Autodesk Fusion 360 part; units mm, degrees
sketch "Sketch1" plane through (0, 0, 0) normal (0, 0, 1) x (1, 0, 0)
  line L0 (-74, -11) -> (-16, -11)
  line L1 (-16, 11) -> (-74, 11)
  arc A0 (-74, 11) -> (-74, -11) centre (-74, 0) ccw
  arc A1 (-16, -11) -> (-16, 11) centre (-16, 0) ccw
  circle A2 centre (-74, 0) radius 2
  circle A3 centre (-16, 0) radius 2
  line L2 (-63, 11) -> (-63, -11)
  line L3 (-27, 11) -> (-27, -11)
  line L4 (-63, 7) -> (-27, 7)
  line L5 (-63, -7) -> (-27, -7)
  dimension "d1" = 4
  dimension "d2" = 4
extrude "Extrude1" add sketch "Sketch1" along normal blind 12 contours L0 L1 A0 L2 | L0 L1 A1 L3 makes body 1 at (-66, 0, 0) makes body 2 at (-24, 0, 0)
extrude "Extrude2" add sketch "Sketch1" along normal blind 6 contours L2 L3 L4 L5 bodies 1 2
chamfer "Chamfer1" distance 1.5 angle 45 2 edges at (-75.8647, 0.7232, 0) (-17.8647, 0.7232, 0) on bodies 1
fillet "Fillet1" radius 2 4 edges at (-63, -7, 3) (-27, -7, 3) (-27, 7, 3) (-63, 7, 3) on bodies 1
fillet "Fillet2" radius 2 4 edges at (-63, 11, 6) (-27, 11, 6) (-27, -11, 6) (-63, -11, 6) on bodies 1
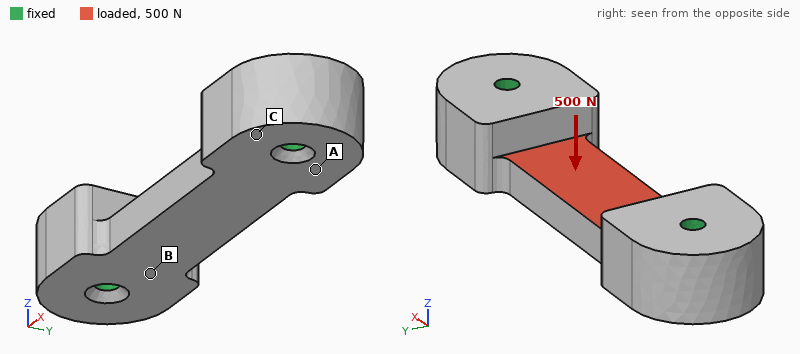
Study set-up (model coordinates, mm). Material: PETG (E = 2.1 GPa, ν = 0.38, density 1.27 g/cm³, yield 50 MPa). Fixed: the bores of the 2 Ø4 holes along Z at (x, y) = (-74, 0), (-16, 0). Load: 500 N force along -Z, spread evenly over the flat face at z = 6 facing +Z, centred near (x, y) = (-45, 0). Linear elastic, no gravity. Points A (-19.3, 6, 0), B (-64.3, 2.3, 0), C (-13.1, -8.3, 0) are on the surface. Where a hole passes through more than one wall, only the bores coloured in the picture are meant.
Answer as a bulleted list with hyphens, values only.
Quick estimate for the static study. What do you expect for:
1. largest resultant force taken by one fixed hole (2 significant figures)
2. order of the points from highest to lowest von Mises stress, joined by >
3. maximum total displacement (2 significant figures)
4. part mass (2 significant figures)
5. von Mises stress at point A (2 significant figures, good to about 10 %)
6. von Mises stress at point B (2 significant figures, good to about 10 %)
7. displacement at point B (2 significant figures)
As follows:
- 280 N
- B > A > C
- 0.32 mm
- 17 g
- 3.8 MPa
- 8.3 MPa
- 0.075 mm
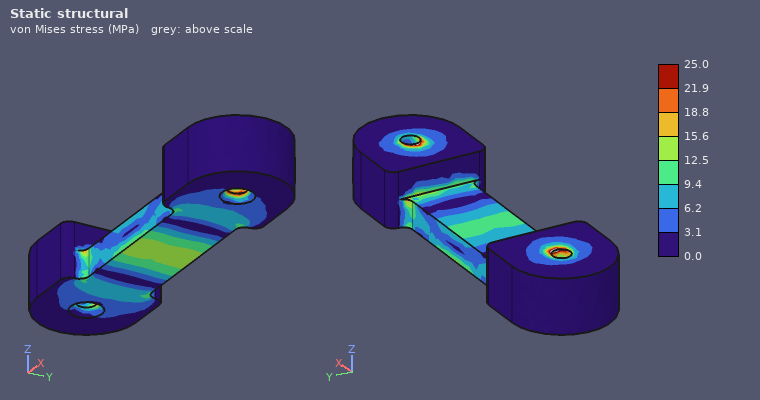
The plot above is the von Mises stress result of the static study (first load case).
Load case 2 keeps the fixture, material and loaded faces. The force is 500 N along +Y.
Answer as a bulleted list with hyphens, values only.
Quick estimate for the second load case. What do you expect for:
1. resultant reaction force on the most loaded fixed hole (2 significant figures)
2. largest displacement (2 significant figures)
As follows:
- 250 N
- 0.27 mm
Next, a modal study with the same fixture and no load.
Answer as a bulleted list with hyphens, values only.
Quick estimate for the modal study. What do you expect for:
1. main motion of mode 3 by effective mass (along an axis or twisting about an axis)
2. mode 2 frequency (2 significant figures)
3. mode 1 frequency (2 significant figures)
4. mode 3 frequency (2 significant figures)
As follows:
- twisting about X
- 3500 Hz
- 3500 Hz
- 6500 Hz
